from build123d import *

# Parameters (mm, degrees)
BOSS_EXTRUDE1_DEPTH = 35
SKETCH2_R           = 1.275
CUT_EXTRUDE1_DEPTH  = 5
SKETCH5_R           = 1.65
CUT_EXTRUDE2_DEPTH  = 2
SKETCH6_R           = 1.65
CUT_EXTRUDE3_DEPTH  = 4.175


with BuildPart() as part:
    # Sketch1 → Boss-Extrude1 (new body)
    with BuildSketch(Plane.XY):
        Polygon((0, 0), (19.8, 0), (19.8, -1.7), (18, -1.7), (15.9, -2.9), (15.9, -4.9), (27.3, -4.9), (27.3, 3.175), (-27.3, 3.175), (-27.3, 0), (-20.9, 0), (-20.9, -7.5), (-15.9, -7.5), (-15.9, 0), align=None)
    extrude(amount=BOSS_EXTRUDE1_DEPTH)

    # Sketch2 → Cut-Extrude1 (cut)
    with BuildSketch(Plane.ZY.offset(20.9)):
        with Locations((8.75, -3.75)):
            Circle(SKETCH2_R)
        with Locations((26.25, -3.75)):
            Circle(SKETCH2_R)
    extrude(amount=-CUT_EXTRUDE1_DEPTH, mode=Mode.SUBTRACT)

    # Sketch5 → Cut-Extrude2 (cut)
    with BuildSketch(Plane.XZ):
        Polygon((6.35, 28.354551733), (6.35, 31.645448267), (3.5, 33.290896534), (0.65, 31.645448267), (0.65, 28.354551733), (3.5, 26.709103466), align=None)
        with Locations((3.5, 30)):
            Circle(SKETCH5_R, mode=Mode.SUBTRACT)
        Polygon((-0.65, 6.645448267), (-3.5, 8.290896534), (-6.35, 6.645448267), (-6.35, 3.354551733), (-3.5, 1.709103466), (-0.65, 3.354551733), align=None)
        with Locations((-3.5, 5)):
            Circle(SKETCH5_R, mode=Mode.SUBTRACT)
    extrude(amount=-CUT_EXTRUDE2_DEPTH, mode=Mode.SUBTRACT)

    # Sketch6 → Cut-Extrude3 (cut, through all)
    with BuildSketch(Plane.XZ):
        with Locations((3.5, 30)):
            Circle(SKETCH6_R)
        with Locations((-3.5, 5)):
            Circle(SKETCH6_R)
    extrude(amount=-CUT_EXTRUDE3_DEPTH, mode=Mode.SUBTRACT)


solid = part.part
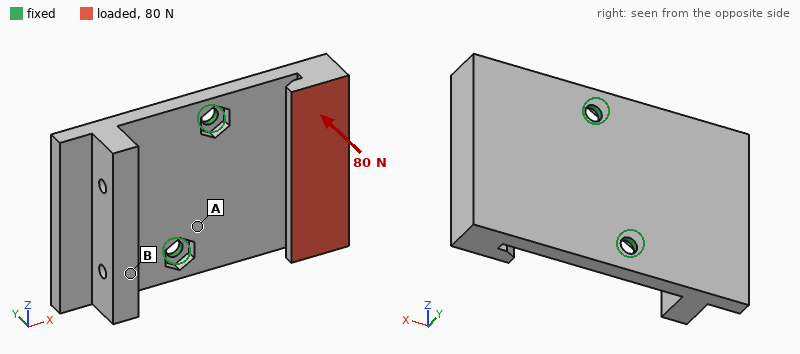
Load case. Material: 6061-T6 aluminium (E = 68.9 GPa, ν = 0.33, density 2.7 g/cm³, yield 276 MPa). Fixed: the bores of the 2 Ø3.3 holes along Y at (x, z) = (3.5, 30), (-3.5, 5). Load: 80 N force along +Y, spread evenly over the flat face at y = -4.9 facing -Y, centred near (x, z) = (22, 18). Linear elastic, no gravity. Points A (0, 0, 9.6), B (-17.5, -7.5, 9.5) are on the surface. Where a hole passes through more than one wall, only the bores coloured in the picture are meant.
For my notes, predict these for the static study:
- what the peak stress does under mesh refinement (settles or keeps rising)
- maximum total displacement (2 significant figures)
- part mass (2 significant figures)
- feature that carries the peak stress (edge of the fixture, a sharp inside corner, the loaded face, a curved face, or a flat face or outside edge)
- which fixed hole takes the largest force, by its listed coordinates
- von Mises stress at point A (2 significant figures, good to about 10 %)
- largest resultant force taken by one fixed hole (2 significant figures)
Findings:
keeps rising
0.15 mm
24 g
edge of the fixture
(3.5, 30)
28 MPa
68 N
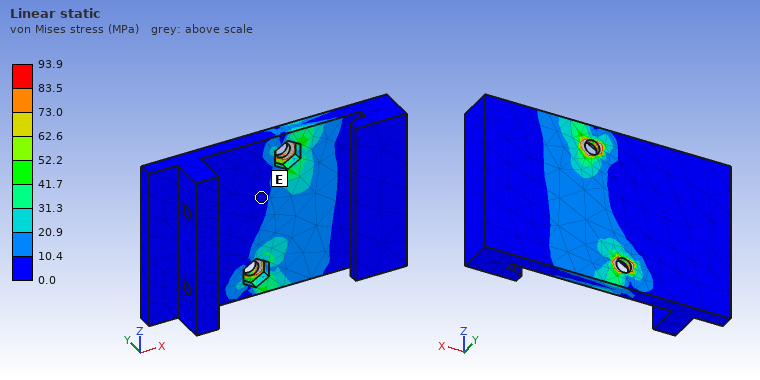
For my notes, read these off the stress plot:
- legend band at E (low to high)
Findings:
0.0 to 10.4 MPa
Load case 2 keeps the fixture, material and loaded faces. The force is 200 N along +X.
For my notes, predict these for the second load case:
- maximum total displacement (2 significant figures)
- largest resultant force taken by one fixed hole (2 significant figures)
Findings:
0.15 mm
100 N
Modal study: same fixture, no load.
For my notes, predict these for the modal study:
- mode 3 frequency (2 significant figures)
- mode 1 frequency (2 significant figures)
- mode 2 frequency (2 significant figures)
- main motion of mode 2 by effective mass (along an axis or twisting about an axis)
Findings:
4700 Hz
1300 Hz
2400 Hz
along Y
